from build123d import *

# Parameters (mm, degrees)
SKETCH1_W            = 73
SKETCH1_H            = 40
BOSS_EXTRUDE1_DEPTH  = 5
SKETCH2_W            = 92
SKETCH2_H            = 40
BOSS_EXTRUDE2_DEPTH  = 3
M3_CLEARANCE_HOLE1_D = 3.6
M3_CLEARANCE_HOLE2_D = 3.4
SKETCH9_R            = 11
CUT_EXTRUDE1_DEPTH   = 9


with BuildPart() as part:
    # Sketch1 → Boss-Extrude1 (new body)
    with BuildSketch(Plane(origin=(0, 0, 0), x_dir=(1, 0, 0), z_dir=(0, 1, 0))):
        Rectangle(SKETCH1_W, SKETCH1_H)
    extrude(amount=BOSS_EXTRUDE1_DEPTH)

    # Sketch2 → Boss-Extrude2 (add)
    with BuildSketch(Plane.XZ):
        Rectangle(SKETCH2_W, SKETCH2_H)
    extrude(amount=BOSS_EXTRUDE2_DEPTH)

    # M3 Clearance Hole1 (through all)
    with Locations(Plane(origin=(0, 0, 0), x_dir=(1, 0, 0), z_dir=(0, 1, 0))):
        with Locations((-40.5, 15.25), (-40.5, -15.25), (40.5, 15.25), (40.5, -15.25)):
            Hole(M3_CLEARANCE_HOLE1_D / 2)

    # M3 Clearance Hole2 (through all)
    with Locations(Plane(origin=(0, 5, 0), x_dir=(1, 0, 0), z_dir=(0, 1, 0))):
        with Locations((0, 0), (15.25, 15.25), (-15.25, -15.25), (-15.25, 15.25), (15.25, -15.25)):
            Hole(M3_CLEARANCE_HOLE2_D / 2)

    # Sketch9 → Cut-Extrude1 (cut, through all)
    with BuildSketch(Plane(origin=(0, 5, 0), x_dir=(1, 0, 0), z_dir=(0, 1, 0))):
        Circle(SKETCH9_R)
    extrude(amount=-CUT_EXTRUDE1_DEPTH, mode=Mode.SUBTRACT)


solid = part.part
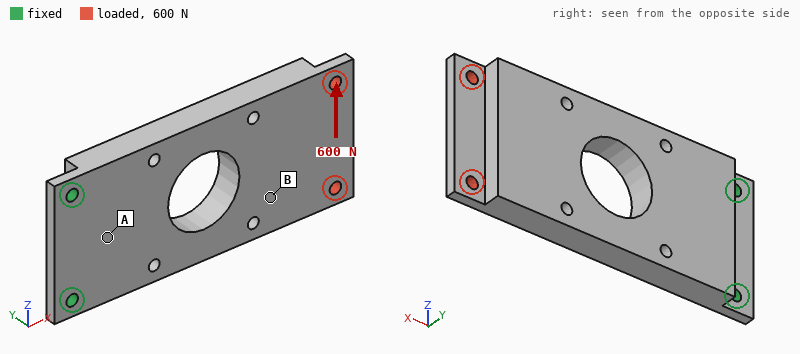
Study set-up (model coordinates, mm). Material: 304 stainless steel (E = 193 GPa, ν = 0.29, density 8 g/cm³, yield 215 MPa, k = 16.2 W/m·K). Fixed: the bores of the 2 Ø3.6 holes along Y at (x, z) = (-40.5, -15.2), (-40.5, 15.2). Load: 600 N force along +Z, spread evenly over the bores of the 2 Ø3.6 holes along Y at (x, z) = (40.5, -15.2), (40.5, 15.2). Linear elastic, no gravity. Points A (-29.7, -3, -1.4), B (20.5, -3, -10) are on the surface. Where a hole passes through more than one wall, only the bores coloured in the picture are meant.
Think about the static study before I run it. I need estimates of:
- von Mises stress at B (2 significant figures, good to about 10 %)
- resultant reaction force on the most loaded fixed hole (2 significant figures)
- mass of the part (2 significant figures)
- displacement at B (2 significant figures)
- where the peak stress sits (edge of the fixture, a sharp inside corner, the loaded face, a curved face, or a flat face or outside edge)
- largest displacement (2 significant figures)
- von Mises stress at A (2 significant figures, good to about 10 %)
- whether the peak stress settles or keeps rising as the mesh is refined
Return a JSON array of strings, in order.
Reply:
["8.9 MPa", "1.6 kN", "180 g", "25 µm", "edge of the fixture", "38 µm", "22 MPa", "keeps rising"]
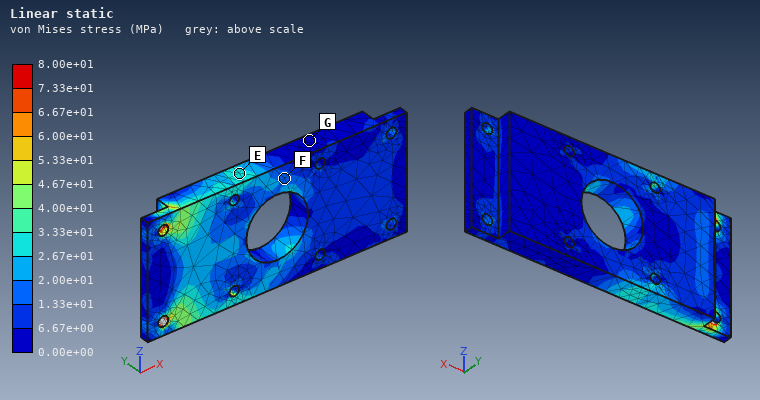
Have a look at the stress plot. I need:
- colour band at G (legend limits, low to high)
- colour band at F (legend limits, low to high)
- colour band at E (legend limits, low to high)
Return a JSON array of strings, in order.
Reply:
["0.00e+00 to 6.67e+00 MPa", "1.33e+01 to 2.00e+01 MPa", "2.67e+01 to 3.33e+01 MPa"]
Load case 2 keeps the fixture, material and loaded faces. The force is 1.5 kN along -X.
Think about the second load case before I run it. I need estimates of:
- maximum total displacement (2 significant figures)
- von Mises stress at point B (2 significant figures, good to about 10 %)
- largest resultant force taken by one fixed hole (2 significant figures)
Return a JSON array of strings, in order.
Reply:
["57 µm", "15 MPa", "760 N"]
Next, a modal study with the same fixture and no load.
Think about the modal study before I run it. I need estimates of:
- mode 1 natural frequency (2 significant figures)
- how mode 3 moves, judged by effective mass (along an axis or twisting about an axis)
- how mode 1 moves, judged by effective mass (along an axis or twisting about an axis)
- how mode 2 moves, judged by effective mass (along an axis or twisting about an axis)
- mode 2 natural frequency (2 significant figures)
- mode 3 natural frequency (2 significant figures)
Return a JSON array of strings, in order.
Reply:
["400 Hz", "along Z", "along Y", "along Z", "2700 Hz", "3400 Hz"]
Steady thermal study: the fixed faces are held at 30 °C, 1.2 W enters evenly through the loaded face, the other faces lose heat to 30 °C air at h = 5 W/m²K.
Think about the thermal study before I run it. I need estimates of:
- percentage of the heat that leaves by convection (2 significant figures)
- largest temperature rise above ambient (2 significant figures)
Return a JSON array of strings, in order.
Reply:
["42 %", "26 K"]
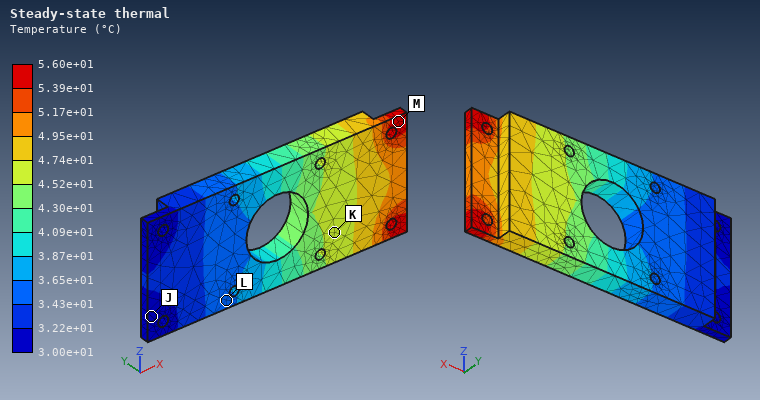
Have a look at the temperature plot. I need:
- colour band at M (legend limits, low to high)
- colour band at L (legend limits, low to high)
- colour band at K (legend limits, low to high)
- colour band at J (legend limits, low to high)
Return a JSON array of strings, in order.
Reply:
["5.39e+01 to 5.60e+01 °C", "3.43e+01 to 3.65e+01 °C", "4.52e+01 to 4.74e+01 °C", "3.00e+01 to 3.22e+01 °C"]
